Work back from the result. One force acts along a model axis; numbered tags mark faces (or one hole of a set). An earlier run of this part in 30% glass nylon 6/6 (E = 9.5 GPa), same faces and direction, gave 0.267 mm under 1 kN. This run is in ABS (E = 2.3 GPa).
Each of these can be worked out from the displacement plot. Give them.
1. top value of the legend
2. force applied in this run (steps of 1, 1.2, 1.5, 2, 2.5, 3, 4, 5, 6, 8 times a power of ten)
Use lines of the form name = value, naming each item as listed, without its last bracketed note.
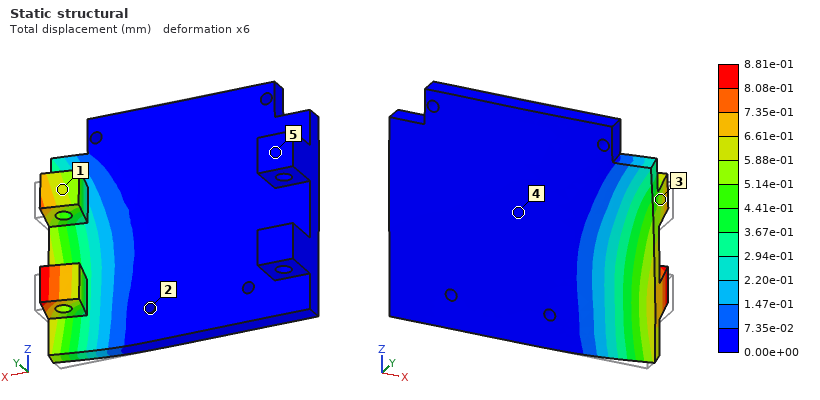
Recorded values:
top value of the legend = 8.81e-01 mm
force applied in this run = 800 N
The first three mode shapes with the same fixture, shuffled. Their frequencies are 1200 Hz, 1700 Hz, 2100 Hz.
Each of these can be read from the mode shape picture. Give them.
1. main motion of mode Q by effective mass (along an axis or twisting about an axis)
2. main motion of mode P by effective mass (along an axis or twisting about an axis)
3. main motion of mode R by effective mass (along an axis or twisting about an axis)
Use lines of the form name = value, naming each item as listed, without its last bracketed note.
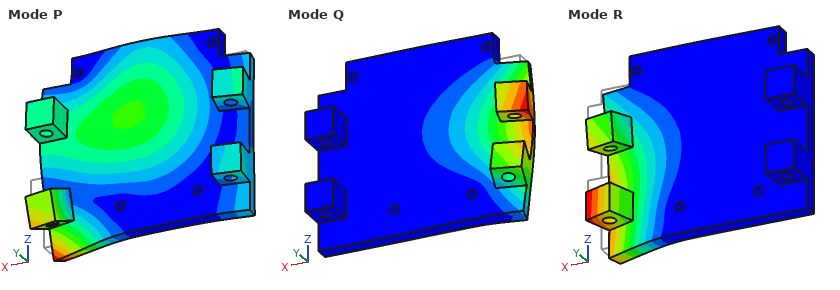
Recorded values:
main motion of mode Q by effective mass = along Y
main motion of mode P by effective mass = along Y
main motion of mode R by effective mass = along Y
